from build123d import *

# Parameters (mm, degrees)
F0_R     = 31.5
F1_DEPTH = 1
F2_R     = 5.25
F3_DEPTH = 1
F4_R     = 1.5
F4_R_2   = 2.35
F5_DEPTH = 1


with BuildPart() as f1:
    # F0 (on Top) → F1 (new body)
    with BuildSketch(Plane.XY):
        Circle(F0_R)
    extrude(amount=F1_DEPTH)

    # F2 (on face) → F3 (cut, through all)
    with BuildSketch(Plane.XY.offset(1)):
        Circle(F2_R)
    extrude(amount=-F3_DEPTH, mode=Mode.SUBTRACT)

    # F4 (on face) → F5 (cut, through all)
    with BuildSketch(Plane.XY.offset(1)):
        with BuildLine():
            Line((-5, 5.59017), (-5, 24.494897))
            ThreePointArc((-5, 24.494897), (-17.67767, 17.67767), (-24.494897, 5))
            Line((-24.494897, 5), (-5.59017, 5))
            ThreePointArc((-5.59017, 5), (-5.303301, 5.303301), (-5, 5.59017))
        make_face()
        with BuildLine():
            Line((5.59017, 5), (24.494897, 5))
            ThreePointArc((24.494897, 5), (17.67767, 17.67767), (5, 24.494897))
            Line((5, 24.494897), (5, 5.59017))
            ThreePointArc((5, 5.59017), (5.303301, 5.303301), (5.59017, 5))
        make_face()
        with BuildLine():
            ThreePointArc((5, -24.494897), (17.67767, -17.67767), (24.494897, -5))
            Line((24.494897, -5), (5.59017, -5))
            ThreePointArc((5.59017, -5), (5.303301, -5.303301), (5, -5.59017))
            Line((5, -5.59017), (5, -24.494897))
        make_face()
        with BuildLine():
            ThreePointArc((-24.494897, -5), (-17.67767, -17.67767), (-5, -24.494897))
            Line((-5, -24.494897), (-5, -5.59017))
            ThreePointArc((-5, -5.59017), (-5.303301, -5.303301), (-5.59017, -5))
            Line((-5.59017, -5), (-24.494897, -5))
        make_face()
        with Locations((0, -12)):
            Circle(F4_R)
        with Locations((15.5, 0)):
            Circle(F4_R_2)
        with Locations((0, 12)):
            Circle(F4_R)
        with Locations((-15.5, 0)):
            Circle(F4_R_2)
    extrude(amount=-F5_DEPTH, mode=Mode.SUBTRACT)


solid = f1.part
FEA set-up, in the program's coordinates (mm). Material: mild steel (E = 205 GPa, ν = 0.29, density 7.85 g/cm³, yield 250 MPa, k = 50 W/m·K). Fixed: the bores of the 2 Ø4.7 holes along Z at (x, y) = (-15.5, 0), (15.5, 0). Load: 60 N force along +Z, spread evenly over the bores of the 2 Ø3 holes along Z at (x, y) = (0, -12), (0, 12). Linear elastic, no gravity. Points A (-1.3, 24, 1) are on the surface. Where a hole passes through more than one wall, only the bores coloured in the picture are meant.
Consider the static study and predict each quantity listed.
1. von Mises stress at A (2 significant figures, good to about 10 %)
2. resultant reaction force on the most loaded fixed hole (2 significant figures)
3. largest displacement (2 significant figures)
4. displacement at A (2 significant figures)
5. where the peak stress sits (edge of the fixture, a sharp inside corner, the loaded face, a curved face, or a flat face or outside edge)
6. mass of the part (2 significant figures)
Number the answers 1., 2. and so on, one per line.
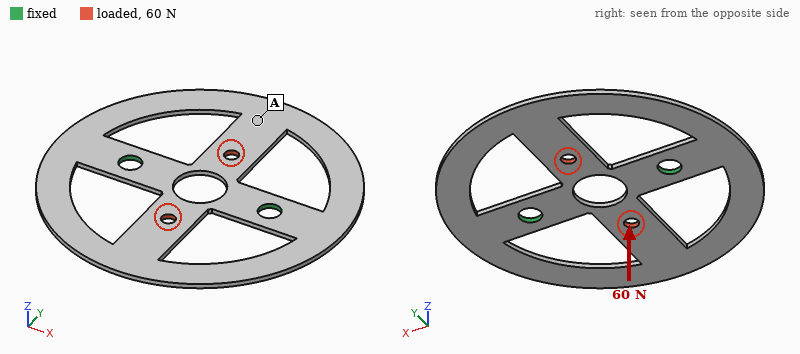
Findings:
1. 21 MPa
2. 30 N
3. 0.21 mm
4. 0.16 mm
5. a flat face or outside edge
6. 15 g
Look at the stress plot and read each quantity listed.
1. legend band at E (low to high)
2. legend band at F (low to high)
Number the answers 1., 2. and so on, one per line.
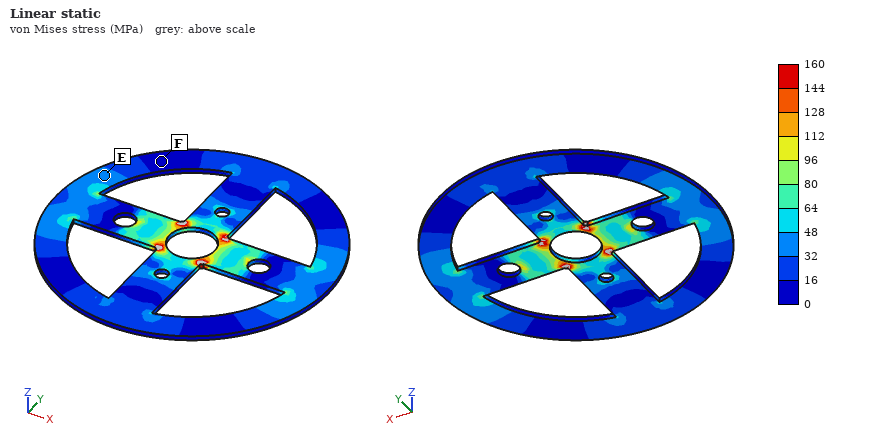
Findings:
1. 32 to 48 MPa
2. 0 to 16 MPa
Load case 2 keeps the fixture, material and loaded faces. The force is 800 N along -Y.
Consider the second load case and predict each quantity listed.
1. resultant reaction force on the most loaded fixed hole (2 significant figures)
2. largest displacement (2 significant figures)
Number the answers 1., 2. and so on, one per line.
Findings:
1. 400 N
2. 10 µm
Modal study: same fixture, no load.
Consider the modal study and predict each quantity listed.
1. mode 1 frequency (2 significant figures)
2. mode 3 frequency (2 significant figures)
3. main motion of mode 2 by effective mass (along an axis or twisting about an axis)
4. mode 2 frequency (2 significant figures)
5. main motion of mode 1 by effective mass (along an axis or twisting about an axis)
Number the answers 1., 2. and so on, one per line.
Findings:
1. 620 Hz
2. 1500 Hz
3. along Z
4. 720 Hz
5. twisting about X
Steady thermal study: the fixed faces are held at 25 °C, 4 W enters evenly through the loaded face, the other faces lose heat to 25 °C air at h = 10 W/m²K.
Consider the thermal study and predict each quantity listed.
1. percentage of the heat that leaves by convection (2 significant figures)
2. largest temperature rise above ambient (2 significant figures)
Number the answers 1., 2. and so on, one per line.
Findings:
1. 24 %
2. 54 K
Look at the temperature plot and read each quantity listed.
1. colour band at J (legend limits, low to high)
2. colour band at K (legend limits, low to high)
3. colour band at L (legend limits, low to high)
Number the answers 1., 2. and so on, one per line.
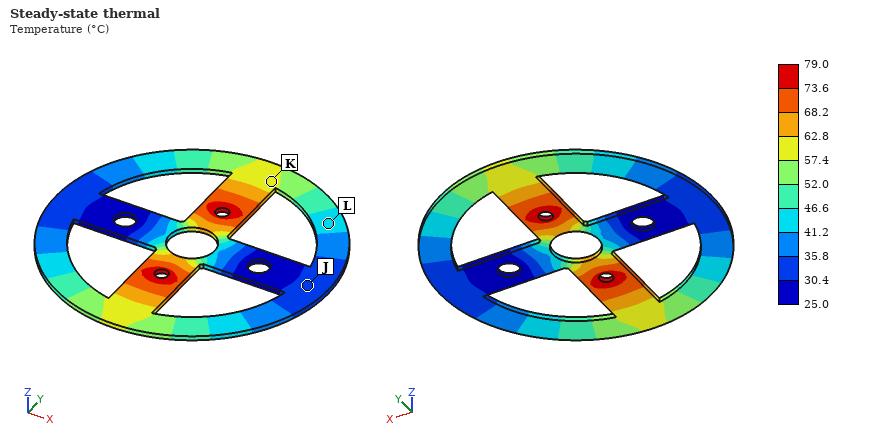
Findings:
1. 30.4 to 35.8 °C
2. 57.4 to 62.8 °C
3. 41.2 to 46.6 °C
